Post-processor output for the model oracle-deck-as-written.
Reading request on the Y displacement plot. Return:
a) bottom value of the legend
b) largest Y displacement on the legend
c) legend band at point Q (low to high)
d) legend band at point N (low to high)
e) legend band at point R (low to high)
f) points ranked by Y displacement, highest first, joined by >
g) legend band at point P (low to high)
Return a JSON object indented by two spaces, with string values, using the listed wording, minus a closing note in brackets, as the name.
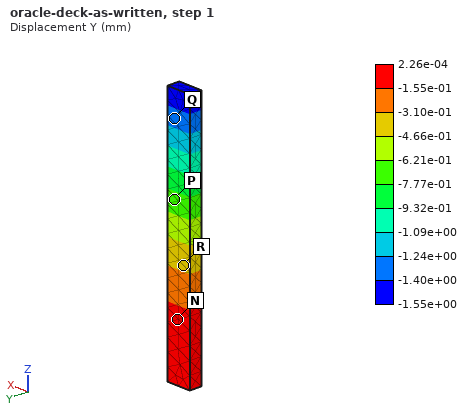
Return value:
{
  "bottom value of the legend": "-1.55e+00 mm",
  "largest Y displacement on the legend": "2.26e-04 mm",
  "legend band at point Q": "-1.40e+00 to -1.24e+00 mm",
  "legend band at point N": "-1.55e-01 to 2.26e-04 mm",
  "legend band at point R": "-4.66e-01 to -3.10e-01 mm",
  "points ranked by Y displacement, highest first, joined by >": "N > R > P > Q",
  "legend band at point P": "-7.77e-01 to -6.21e-01 mm"
}
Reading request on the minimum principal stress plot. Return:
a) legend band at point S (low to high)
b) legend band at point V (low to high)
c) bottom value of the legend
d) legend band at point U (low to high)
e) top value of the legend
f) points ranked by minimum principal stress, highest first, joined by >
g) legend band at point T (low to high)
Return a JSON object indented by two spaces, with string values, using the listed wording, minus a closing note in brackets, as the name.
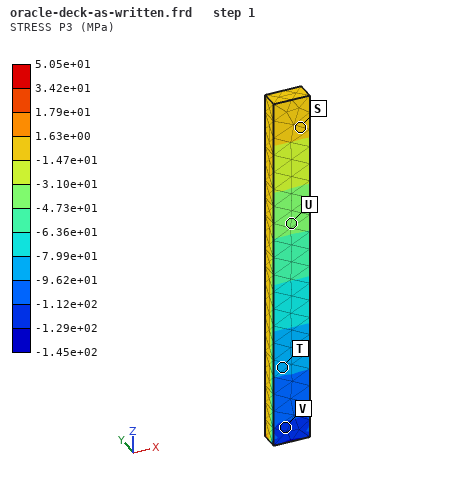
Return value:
{
  "legend band at point S": "-1.47e+01 to 1.63e+00 MPa",
  "legend band at point V": "-1.29e+02 to -1.12e+02 MPa",
  "bottom value of the legend": "-1.45e+02 MPa",
  "legend band at point U": "-4.73e+01 to -3.10e+01 MPa",
  "top value of the legend": "5.05e+01 MPa",
  "points ranked by minimum principal stress, highest first, joined by >": "S > U > T > V",
  "legend band at point T": "-9.62e+01 to -7.99e+01 MPa"
}
